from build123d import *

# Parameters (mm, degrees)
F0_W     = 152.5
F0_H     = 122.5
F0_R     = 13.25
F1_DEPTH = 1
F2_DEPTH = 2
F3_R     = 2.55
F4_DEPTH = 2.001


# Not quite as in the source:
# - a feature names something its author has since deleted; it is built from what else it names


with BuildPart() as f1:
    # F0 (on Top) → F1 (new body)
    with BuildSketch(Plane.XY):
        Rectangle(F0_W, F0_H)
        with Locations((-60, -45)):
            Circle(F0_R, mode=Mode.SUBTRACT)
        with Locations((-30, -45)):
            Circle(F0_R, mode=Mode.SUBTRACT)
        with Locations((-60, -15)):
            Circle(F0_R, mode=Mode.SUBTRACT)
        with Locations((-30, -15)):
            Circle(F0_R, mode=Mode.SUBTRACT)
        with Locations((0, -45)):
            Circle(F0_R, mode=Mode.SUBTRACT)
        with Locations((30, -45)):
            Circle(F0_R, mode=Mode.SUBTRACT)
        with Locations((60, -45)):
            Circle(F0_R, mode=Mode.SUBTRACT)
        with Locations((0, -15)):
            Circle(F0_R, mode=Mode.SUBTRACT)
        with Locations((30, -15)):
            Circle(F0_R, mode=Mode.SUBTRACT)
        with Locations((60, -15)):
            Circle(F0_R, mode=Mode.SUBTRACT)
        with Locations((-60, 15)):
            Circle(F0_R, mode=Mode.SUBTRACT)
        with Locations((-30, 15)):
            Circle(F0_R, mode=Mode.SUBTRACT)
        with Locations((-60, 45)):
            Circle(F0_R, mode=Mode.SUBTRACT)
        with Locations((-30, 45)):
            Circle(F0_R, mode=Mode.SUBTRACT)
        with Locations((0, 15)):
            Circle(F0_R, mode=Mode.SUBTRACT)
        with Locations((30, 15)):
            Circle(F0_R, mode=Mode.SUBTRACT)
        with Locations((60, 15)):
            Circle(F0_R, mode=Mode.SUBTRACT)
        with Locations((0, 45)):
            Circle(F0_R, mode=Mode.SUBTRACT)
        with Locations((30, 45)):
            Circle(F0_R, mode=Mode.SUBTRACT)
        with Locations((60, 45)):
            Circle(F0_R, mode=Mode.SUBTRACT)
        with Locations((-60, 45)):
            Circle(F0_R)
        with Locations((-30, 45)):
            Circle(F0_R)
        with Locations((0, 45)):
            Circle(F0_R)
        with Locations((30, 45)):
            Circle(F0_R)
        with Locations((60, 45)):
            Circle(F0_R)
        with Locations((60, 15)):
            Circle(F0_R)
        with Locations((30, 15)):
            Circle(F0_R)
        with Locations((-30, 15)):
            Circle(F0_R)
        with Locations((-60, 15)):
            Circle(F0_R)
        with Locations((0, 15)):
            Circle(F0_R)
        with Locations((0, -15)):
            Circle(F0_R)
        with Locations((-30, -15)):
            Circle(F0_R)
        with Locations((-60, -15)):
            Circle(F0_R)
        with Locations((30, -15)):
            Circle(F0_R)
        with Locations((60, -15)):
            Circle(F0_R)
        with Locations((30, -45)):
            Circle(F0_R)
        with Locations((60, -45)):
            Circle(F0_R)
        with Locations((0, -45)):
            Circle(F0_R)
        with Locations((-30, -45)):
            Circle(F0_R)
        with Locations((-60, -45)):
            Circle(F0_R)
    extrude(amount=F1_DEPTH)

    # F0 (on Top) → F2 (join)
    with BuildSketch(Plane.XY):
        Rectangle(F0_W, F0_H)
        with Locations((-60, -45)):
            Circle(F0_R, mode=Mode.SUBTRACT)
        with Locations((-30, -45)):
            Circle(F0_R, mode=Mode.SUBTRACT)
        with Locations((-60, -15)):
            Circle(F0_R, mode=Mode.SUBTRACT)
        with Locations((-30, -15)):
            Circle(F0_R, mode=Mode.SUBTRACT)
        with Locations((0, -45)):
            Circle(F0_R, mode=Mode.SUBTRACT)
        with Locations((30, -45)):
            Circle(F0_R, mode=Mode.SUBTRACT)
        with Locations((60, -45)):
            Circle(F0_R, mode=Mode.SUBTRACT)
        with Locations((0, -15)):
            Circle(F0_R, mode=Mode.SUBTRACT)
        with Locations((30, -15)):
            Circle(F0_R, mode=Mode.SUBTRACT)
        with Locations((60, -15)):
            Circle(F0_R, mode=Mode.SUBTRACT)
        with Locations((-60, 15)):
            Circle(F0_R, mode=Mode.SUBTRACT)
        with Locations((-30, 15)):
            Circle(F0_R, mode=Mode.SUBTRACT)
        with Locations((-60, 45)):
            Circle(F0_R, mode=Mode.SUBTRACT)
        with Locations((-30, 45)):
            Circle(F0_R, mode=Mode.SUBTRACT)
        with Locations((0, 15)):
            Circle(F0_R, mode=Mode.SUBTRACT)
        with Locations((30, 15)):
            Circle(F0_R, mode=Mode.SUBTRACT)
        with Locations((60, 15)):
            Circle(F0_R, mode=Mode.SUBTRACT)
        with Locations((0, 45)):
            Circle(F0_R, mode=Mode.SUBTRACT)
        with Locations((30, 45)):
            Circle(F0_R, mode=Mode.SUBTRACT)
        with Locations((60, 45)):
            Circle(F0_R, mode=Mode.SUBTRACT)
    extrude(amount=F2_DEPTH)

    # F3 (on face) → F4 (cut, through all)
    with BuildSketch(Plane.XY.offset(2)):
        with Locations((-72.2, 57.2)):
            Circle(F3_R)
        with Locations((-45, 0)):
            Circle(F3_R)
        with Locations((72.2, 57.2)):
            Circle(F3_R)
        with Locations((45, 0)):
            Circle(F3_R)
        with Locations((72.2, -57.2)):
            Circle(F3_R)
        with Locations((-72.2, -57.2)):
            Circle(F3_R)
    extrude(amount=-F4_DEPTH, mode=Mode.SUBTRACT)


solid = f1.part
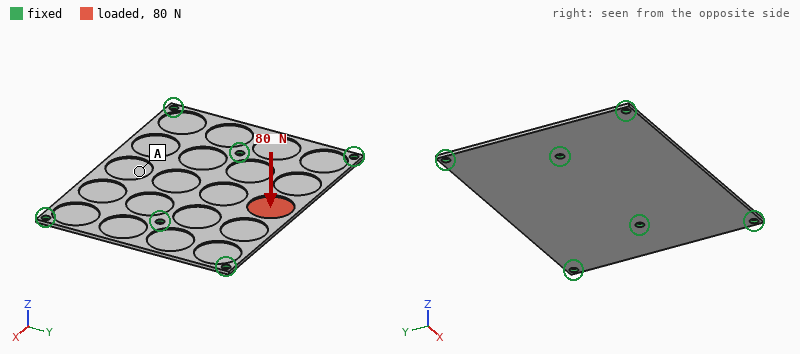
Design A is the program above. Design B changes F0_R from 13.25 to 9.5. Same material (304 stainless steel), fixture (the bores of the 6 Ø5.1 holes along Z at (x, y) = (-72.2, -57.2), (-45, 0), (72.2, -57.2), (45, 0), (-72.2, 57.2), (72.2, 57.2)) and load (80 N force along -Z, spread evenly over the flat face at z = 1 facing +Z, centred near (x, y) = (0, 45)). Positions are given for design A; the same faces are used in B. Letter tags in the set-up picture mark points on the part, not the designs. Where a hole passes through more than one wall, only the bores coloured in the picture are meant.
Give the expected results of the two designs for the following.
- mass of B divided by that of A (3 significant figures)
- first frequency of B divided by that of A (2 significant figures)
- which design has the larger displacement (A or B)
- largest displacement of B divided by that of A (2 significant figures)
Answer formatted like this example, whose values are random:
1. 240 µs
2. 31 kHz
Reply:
1. 1.21
2. 1.1
3. A
4. 0.65
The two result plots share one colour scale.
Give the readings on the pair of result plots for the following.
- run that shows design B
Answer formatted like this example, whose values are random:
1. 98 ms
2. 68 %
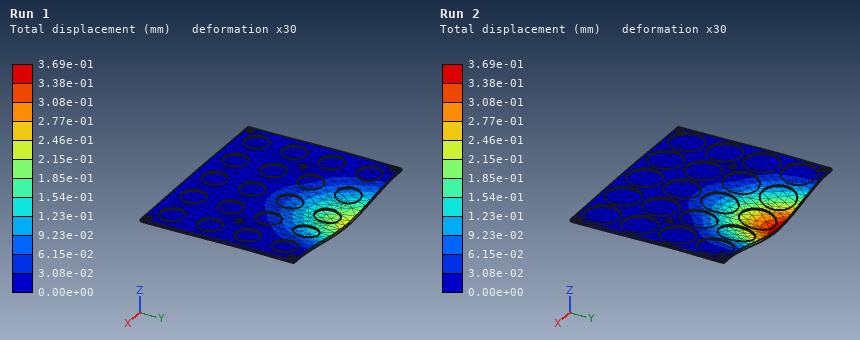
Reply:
1. Run 1
